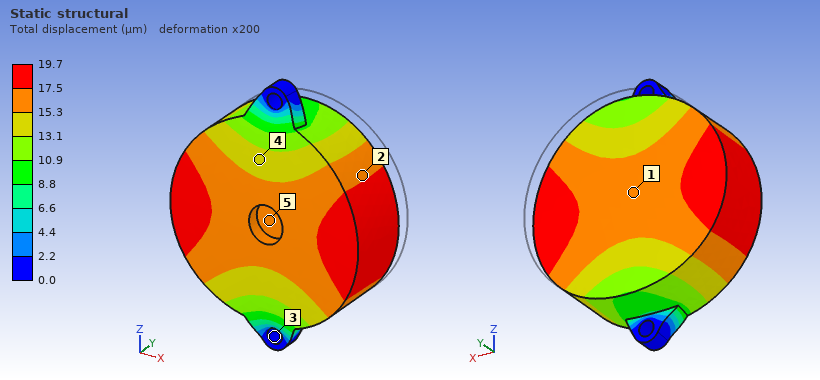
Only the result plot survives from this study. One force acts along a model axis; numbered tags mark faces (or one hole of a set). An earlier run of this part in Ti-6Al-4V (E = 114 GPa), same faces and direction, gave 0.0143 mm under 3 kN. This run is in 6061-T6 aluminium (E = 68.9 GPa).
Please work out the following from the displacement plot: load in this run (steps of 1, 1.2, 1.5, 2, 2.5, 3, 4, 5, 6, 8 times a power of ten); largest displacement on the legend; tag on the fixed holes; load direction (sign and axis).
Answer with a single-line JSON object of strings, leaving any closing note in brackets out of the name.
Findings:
{"load in this run": "2.5 kN", "largest displacement on the legend": "19.7 µm", "tag on the fixed holes": "3", "load direction": "-Y"}
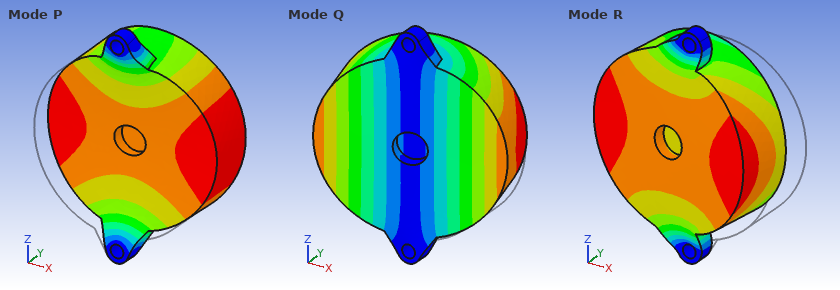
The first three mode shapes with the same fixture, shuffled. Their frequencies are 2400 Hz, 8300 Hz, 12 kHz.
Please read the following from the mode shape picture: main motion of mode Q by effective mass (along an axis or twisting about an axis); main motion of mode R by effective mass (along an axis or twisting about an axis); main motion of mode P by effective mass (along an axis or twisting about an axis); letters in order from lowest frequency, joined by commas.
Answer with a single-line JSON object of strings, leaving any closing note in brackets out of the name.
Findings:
{"main motion of mode Q by effective mass": "along X", "main motion of mode R by effective mass": "along X", "main motion of mode P by effective mass": "along Y", "letters in order from lowest frequency, joined by commas": "Q, P, R"}
